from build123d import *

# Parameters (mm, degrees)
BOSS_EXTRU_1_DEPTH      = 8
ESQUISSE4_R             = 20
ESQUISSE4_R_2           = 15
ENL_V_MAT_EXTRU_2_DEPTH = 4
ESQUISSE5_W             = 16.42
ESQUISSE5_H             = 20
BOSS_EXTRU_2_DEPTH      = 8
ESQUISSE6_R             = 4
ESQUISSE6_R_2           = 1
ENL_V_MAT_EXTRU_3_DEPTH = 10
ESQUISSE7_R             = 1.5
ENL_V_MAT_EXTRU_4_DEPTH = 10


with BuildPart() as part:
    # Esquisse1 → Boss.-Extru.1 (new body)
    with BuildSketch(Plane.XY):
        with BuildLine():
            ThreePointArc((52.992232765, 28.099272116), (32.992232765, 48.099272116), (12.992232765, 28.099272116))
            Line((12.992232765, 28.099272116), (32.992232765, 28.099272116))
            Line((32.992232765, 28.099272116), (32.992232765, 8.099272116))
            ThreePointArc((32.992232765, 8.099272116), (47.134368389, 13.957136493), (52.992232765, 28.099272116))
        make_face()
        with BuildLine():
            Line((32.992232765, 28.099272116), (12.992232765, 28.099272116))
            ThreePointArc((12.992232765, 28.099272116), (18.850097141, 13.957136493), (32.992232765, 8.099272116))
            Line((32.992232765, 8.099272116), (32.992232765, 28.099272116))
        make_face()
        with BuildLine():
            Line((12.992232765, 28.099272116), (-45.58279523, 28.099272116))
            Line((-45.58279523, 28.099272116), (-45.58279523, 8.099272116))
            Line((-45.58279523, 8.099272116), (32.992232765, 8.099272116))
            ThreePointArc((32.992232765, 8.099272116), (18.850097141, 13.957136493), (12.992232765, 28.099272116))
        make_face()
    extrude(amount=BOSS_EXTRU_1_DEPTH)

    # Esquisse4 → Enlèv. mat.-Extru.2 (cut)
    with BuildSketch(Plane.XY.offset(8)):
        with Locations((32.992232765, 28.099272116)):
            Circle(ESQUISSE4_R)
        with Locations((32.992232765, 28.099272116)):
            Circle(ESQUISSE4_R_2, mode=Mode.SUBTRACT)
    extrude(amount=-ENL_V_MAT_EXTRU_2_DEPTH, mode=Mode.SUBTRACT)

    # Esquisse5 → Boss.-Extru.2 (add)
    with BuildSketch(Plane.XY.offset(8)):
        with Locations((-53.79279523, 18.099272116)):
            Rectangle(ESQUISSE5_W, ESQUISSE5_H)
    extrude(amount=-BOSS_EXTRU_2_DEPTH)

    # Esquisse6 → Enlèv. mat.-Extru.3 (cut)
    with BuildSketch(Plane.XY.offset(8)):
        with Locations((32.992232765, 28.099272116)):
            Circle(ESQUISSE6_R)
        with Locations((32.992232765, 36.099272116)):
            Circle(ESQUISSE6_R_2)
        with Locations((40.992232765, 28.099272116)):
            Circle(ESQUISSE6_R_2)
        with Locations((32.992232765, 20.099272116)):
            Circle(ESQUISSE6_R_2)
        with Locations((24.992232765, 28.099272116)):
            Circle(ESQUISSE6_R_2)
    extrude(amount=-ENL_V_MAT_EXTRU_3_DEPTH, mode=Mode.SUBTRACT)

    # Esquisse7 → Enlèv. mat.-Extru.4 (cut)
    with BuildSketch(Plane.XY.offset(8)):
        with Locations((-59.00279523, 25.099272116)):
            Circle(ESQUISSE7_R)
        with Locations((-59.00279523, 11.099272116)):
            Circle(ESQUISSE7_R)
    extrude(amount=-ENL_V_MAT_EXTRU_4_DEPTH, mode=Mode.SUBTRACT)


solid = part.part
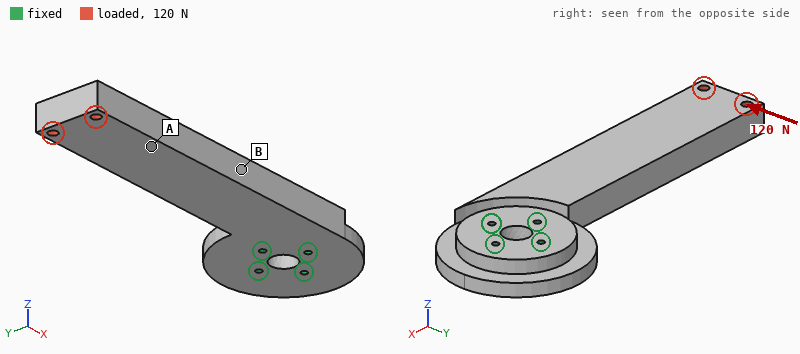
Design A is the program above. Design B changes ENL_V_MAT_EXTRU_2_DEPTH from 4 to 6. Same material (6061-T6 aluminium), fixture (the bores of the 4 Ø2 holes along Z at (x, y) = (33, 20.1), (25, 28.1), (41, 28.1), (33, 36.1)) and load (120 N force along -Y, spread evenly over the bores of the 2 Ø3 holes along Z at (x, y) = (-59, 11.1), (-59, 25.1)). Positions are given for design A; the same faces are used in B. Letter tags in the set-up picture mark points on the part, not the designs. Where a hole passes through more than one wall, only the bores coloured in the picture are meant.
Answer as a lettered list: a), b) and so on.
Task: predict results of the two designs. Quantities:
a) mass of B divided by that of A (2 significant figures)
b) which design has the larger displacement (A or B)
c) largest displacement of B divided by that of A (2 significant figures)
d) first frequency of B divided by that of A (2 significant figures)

a) 0.94
b) B
c) 1.8
d) 0.55
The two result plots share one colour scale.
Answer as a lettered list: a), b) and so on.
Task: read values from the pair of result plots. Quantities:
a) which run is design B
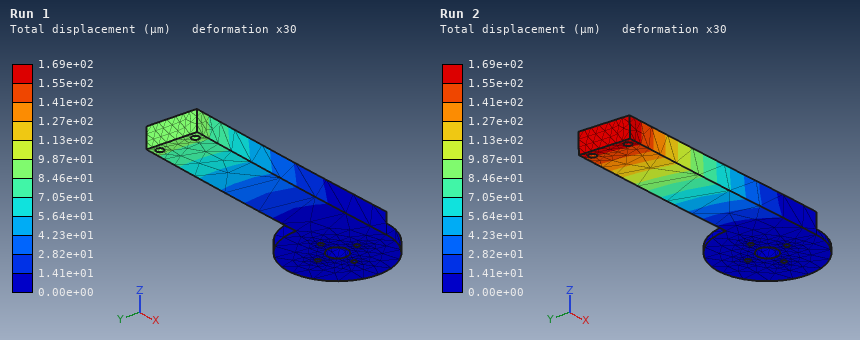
a) Run 2
